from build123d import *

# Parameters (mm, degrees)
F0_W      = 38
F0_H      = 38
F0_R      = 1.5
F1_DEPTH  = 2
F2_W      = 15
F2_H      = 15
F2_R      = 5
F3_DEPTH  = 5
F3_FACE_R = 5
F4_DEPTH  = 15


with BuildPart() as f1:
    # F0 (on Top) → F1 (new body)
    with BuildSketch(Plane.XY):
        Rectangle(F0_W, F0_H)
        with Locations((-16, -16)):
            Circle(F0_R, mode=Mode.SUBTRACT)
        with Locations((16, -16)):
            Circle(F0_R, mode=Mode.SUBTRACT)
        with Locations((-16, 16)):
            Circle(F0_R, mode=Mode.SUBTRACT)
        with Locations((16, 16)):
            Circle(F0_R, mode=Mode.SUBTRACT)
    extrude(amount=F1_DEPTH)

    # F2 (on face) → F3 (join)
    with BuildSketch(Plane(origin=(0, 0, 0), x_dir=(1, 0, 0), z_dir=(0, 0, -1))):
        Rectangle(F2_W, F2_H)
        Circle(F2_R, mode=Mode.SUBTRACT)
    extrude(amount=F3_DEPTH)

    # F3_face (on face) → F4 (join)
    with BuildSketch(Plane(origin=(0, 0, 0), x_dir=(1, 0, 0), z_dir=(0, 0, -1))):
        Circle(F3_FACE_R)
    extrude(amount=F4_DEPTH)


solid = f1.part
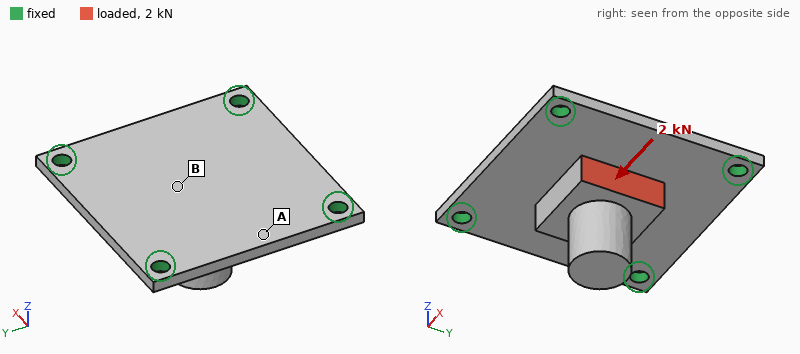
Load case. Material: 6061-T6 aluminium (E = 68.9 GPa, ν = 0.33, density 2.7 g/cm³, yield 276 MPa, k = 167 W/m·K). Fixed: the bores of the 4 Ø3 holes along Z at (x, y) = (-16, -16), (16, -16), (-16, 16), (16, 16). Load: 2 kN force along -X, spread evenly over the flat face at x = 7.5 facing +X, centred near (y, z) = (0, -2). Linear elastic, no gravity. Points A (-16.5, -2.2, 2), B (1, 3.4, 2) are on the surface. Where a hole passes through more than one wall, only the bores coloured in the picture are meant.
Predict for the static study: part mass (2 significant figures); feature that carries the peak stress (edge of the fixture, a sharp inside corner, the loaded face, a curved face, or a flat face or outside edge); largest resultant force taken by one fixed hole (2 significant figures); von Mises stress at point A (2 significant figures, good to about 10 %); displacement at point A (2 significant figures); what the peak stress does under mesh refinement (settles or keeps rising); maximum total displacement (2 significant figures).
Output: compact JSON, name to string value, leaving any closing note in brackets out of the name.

{"part mass": "13 g", "feature that carries the peak stress": "edge of the fixture", "largest resultant force taken by one fixed hole": "580 N", "von Mises stress at point A": "44 MPa", "displacement at point A": "35 µm", "what the peak stress does under mesh refinement": "keeps rising", "maximum total displacement": "77 µm"}
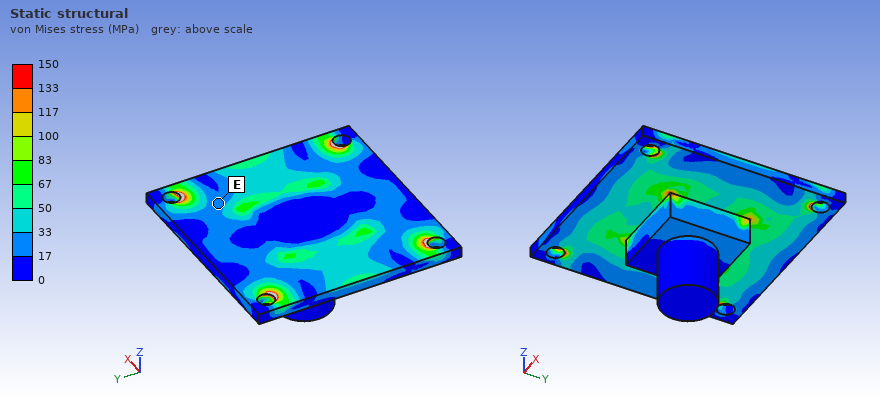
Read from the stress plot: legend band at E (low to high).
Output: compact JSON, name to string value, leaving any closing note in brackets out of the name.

{"legend band at E": "17 to 33 MPa"}
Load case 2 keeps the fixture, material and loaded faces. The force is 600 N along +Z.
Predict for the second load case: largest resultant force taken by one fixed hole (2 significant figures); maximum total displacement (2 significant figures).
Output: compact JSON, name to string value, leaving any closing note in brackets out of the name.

{"largest resultant force taken by one fixed hole": "240 N", "maximum total displacement": "81 µm"}
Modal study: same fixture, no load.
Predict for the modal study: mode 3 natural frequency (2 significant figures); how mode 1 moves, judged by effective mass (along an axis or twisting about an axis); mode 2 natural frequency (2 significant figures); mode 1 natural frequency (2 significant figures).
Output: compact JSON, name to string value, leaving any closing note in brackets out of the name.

{"mode 3 natural frequency": "8300 Hz", "how mode 1 moves, judged by effective mass": "along Z", "mode 2 natural frequency": "8300 Hz", "mode 1 natural frequency": "5600 Hz"}
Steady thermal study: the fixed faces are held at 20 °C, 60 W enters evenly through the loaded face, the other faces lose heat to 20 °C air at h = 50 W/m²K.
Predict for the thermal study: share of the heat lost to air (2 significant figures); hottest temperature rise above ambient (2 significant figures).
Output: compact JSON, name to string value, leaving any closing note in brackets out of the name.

{"share of the heat lost to air": "9.1 %", "hottest temperature rise above ambient": "67 K"}
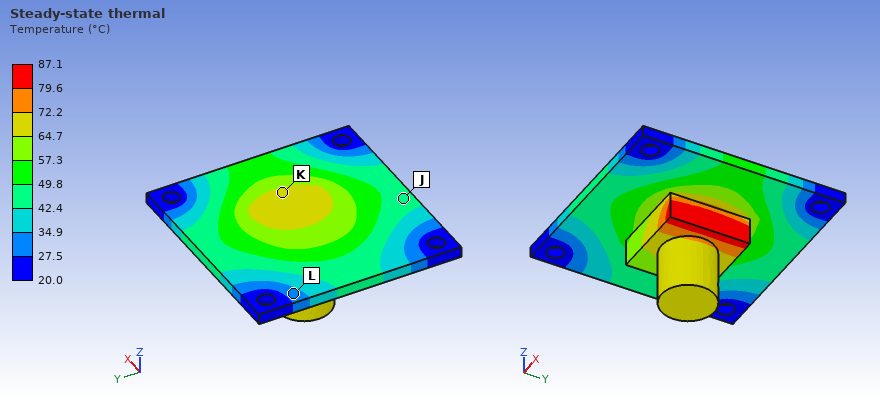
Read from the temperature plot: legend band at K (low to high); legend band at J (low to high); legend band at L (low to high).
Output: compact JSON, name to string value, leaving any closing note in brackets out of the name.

{"legend band at K": "64.7 to 72.2 °C", "legend band at J": "42.4 to 49.8 °C", "legend band at L": "27.5 to 34.9 °C"}
